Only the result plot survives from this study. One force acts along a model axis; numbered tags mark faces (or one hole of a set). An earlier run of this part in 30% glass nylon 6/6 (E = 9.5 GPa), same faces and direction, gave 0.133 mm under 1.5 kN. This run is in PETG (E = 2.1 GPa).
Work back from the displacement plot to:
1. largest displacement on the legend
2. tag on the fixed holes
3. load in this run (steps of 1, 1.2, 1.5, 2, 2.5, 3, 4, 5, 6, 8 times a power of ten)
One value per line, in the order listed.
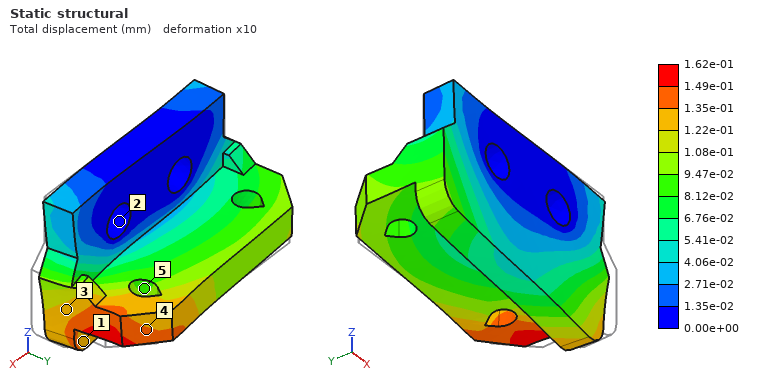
1.62e-01 mm
2
400 N
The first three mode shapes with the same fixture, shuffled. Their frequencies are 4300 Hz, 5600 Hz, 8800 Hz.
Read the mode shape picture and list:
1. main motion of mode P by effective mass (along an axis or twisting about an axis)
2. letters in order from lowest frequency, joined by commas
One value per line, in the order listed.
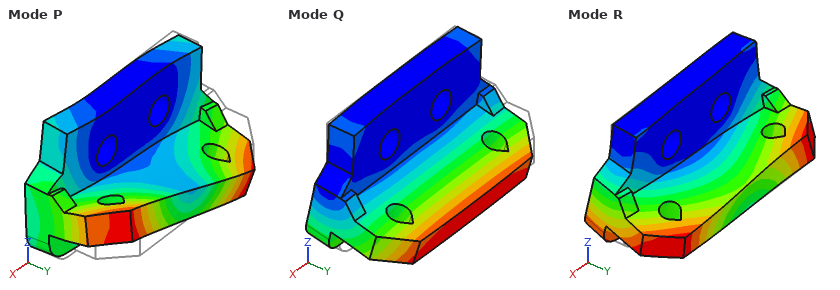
along X
Q, R, P
